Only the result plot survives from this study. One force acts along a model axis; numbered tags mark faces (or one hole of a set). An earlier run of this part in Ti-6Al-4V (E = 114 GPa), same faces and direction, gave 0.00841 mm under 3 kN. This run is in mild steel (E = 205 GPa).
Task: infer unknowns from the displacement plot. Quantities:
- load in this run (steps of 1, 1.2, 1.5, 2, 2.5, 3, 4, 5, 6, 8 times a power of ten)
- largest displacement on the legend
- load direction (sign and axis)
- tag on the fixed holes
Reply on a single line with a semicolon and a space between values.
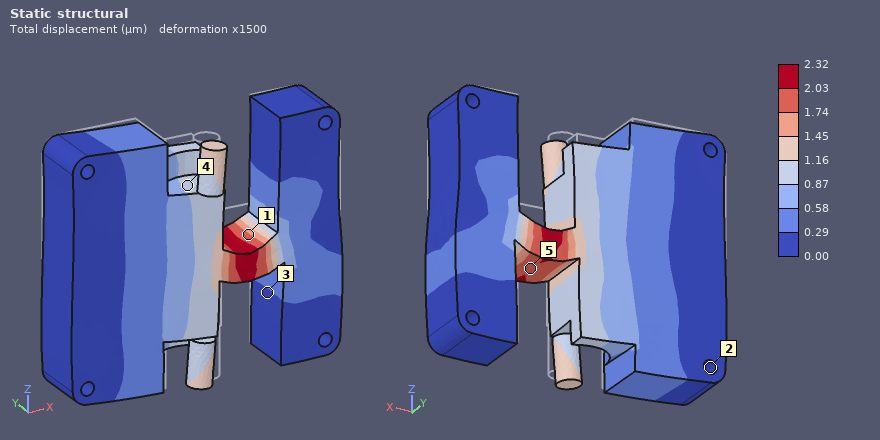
1.5 kN; 2.32 µm; -Z; 2
